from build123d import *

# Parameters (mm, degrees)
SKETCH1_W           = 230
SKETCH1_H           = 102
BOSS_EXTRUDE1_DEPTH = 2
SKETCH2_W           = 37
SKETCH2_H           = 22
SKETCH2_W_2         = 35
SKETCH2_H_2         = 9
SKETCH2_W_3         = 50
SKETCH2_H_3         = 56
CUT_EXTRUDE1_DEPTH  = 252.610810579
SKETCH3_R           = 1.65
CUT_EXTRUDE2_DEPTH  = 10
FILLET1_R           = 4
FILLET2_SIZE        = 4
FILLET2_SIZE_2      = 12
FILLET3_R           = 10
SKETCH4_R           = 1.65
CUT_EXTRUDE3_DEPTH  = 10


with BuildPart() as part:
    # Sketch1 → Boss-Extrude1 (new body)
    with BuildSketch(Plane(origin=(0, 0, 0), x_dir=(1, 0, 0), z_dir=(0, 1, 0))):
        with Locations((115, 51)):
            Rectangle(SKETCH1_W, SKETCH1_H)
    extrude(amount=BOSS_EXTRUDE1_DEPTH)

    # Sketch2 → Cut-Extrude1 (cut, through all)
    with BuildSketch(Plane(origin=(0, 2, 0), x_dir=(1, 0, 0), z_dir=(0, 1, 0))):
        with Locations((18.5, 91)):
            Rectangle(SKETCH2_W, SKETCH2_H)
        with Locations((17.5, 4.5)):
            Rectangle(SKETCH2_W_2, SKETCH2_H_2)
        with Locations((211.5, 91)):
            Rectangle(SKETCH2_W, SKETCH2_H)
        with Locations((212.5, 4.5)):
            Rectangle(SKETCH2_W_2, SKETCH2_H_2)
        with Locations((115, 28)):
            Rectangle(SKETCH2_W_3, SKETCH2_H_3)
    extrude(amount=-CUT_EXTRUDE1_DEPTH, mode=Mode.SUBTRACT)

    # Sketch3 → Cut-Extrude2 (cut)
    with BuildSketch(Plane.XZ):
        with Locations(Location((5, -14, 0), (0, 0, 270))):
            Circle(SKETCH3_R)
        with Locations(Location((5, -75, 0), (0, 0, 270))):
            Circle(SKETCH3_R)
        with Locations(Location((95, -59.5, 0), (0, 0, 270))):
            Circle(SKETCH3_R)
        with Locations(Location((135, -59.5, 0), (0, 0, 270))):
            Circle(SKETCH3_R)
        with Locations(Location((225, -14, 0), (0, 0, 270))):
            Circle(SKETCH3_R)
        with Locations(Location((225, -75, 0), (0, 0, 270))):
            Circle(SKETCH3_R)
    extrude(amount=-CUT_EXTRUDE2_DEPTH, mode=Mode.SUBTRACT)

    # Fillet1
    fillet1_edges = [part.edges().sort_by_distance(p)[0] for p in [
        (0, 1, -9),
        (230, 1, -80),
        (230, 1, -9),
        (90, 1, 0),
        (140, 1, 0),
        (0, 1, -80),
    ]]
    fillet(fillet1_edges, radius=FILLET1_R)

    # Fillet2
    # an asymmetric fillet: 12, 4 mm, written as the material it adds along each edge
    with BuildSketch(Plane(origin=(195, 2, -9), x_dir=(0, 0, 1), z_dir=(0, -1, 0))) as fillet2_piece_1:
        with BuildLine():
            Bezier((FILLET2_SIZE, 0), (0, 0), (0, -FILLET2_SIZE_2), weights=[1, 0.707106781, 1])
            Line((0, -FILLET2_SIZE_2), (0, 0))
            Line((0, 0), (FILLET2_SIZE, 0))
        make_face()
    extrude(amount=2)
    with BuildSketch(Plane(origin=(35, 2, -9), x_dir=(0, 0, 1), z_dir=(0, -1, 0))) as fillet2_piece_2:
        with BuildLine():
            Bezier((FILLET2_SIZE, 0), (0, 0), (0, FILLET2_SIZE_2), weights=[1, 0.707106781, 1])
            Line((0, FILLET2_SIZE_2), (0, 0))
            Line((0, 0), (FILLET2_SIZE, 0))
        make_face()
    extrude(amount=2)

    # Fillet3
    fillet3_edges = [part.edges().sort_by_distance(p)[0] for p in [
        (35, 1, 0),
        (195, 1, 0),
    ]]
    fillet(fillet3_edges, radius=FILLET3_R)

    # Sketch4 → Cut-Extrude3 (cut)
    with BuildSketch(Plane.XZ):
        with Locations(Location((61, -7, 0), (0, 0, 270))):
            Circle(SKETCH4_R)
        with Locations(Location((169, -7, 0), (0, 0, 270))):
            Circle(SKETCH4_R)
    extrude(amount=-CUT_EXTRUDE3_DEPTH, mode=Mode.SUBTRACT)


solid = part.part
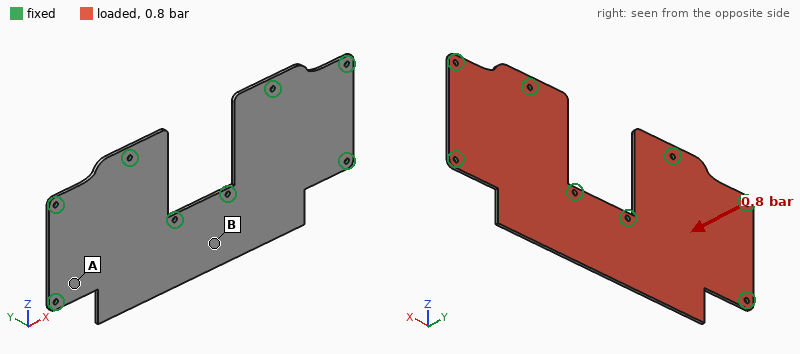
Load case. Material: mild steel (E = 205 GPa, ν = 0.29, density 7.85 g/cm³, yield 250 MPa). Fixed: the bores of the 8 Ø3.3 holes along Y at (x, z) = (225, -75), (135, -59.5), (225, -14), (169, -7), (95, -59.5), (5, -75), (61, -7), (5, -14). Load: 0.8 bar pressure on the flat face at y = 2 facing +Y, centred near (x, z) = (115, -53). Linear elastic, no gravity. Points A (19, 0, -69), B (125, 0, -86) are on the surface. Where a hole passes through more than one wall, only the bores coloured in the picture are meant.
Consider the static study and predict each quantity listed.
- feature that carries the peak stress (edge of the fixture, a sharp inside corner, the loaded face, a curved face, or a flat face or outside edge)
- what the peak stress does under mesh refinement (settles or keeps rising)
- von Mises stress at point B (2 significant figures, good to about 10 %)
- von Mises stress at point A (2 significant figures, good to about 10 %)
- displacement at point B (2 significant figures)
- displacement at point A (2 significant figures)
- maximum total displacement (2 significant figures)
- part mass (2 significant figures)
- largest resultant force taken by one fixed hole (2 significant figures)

edge of the fixture
keeps rising
23 MPa
56 MPa
0.17 mm
0.063 mm
0.40 mm
290 g
310 N
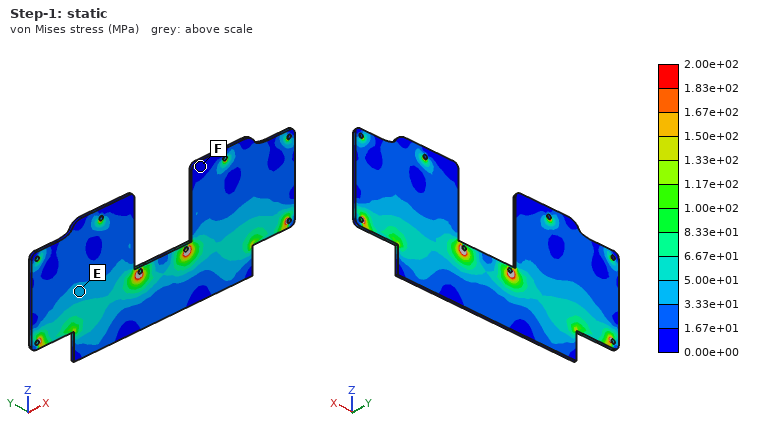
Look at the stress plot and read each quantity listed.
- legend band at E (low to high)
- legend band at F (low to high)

3.33e+01 to 5.00e+01 MPa
0.00e+00 to 1.67e+01 MPa
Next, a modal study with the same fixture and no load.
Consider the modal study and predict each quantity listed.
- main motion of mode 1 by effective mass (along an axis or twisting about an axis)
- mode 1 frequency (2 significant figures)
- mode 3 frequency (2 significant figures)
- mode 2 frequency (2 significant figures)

along Y
730 Hz
1200 Hz
830 Hz
